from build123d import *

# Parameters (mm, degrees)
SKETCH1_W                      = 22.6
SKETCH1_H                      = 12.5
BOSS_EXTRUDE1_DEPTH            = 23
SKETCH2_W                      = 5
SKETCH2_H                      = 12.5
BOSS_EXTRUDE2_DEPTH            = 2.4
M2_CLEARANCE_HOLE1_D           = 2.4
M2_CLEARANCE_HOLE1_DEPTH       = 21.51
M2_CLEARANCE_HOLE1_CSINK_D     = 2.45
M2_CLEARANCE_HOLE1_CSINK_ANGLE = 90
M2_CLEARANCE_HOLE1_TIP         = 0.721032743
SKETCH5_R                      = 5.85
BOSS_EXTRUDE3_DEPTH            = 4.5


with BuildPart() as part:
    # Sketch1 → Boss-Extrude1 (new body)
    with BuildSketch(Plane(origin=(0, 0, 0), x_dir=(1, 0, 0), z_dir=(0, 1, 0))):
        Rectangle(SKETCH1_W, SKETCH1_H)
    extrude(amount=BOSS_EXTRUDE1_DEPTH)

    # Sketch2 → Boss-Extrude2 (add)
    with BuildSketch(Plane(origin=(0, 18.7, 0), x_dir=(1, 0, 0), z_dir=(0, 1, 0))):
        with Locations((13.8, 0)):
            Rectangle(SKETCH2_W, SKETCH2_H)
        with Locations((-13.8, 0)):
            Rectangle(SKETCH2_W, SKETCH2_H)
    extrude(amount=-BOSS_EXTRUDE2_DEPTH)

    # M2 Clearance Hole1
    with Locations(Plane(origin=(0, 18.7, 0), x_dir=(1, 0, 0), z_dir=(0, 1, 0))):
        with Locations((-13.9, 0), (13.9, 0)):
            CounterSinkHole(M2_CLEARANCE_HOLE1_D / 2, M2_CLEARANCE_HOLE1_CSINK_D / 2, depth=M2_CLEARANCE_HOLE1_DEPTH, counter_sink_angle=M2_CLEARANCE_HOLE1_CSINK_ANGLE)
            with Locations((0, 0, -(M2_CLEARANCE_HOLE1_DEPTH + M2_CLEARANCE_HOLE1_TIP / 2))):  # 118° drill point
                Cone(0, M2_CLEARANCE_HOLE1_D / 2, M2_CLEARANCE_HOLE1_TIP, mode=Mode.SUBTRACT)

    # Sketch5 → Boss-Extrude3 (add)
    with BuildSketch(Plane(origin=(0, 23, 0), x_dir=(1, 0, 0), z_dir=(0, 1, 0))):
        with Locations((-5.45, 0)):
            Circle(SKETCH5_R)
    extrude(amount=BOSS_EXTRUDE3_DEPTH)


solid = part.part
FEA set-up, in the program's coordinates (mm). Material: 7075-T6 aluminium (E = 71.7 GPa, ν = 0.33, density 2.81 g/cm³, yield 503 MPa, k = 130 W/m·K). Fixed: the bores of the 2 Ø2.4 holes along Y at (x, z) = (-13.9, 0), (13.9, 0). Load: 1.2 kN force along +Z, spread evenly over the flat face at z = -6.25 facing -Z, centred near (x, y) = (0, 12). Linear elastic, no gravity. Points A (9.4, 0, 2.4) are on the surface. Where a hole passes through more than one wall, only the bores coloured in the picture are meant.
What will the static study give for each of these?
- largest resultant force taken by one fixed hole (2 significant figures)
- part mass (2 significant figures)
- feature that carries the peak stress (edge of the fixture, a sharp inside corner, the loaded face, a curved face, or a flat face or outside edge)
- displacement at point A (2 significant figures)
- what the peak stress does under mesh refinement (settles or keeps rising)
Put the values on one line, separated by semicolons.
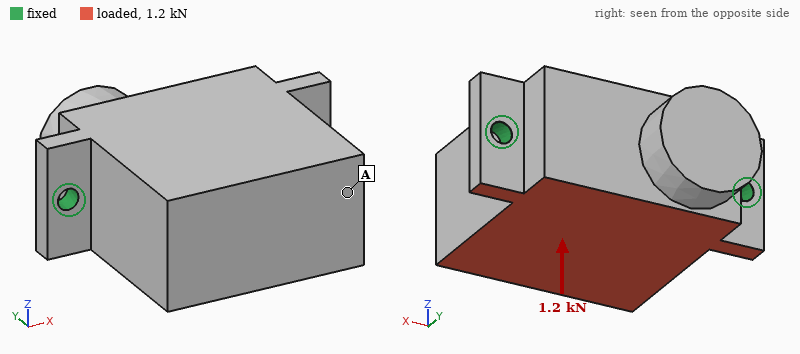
600 N; 20 g; edge of the fixture; 0.12 mm; keeps rising
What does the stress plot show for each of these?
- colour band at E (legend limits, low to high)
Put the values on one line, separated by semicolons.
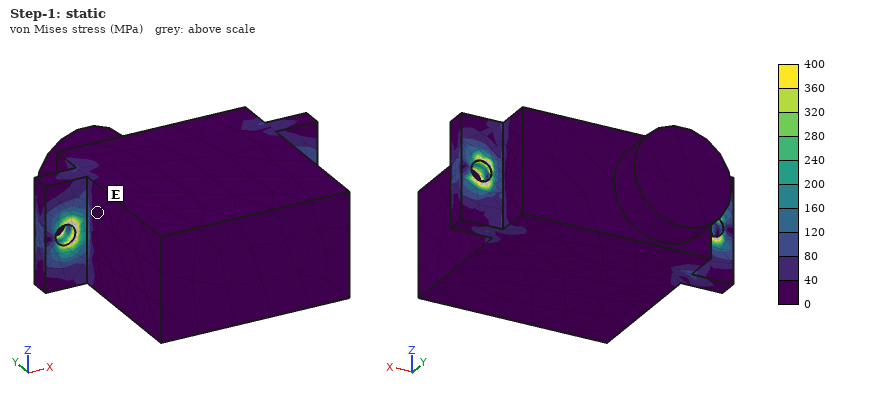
0 to 40 MPa
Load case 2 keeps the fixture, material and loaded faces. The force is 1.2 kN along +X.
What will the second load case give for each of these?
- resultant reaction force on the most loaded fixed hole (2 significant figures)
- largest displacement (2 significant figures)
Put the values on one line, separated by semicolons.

710 N; 10 µm
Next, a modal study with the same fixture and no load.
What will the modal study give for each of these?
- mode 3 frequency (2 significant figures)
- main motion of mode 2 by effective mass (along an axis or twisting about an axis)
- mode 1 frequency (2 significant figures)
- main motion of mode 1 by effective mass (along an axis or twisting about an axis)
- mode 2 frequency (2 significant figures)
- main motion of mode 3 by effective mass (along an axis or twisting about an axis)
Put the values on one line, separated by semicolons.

16 kHz; along Y; 3800 Hz; along Z; 15 kHz; along X
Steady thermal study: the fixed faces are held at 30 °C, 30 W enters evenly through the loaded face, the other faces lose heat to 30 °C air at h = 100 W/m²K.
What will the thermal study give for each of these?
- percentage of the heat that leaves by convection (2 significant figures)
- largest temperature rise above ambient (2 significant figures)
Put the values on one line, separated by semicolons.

11 %; 23 K
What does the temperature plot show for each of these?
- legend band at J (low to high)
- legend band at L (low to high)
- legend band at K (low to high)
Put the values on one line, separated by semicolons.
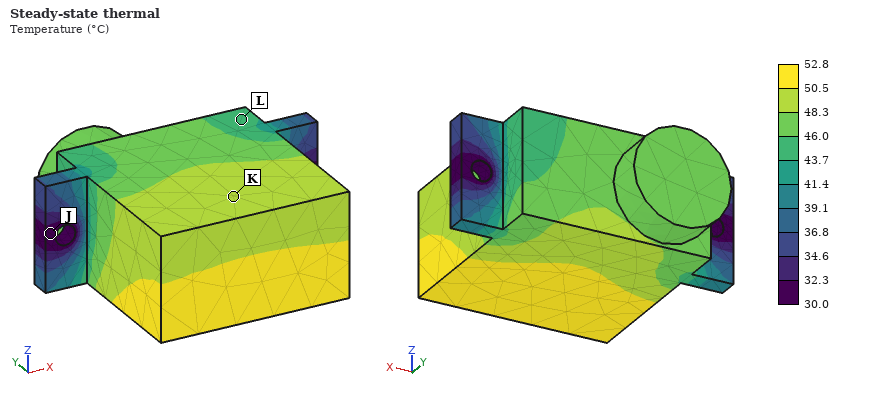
30.0 to 32.3 °C; 43.7 to 46.0 °C; 48.3 to 50.5 °C
